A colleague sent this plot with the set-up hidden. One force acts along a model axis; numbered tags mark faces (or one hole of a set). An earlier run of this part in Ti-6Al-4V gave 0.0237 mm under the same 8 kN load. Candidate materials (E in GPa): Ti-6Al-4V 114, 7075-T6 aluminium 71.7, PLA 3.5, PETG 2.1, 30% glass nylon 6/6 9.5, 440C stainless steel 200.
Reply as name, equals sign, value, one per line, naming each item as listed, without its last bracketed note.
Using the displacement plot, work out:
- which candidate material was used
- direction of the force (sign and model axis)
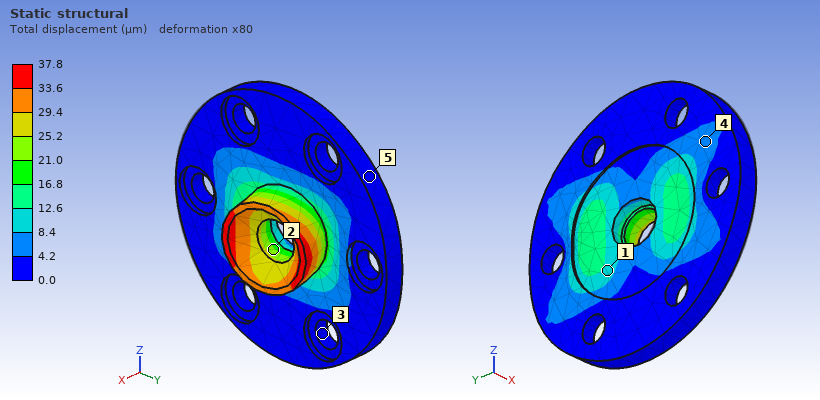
which candidate material was used = 7075-T6 aluminium
direction of the force = +Y
